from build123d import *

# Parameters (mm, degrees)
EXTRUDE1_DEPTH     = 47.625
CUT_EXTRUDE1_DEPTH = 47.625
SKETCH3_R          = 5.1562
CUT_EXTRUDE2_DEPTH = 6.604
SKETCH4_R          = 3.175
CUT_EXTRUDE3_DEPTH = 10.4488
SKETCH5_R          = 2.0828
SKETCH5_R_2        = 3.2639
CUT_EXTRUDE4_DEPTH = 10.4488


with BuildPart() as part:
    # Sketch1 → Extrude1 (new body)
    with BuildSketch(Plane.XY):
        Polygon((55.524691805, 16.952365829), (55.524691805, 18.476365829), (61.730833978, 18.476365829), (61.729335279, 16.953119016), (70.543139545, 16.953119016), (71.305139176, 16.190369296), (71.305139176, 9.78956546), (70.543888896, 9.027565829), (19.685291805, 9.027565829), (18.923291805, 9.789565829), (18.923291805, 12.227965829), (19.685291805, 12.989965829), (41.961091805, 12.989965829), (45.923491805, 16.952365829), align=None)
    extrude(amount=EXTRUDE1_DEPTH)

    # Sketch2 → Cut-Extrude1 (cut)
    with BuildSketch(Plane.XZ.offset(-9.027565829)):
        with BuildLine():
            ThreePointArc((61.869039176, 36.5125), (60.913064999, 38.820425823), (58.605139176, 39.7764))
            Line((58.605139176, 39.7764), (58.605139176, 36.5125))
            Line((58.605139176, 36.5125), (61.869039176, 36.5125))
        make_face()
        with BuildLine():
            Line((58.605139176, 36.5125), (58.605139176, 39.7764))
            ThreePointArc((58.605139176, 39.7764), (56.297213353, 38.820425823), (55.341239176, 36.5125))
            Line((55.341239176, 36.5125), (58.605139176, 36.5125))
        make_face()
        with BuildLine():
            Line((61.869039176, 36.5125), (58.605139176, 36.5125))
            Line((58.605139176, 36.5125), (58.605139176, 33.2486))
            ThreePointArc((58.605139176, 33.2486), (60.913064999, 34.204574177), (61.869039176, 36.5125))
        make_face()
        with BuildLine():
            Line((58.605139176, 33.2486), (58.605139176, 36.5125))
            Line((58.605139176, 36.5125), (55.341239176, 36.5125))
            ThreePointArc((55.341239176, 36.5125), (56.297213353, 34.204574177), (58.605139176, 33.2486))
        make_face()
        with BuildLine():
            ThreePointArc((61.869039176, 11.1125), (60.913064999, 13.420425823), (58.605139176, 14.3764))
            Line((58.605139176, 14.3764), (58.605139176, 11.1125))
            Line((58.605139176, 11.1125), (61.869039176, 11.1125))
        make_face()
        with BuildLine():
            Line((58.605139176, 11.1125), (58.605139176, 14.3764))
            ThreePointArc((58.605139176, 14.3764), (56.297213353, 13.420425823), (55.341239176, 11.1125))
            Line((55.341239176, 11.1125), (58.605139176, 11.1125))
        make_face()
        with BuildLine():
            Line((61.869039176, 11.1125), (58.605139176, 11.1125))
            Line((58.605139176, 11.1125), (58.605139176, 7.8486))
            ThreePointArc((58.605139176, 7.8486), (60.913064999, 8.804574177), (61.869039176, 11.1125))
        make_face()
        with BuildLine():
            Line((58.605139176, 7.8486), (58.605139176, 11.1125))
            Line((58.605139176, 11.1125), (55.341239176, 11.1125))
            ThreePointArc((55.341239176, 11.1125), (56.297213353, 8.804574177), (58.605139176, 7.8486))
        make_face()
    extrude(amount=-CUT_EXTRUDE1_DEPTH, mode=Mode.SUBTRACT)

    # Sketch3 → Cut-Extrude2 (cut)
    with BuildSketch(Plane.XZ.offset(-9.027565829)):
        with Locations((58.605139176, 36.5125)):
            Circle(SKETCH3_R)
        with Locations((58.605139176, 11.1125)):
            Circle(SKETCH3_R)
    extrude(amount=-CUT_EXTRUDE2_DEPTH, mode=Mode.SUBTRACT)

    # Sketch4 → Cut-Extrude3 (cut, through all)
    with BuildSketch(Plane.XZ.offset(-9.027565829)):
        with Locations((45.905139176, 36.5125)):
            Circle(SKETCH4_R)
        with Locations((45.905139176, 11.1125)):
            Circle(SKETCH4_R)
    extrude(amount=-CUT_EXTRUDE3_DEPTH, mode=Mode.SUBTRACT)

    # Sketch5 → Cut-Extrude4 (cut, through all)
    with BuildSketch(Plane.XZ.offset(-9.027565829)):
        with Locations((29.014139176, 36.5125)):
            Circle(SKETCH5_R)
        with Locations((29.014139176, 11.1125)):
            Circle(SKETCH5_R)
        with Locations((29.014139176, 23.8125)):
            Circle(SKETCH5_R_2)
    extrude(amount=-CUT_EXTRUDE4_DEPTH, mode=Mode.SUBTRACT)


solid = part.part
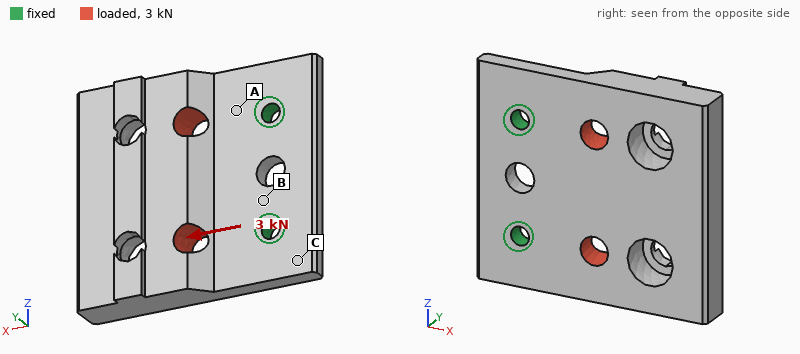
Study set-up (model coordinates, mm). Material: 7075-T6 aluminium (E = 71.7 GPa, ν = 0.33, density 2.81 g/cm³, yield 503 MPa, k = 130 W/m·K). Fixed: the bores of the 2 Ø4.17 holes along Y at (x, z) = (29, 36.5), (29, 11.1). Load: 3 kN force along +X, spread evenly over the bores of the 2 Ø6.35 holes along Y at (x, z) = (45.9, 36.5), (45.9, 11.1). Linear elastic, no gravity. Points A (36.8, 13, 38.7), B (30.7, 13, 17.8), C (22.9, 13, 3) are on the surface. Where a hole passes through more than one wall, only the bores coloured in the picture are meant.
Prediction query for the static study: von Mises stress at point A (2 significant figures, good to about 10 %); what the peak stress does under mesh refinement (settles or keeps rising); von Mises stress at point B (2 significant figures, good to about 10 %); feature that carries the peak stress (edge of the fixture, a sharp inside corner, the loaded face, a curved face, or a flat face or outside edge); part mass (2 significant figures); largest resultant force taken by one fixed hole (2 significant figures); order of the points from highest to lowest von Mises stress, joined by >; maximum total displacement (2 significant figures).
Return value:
59 MPa
keeps rising
39 MPa
edge of the fixture
38 g
1.5 kN
A > B > C
0.15 mm
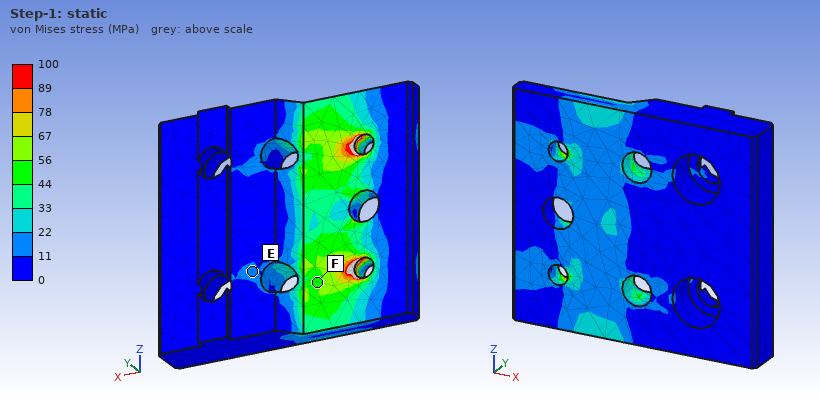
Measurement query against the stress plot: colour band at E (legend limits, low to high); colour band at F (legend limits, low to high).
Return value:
11 to 22 MPa
44 to 56 MPa
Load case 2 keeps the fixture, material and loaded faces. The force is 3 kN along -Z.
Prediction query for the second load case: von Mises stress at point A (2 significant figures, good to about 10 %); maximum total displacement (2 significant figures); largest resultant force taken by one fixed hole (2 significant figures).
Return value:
30 MPa
38 µm
2.3 kN
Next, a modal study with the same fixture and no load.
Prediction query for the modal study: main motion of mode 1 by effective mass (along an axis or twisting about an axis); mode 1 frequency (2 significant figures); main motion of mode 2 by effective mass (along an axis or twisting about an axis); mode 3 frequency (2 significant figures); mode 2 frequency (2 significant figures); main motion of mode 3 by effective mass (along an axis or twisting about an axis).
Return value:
along Y
1400 Hz
twisting about X
7900 Hz
4300 Hz
along Z
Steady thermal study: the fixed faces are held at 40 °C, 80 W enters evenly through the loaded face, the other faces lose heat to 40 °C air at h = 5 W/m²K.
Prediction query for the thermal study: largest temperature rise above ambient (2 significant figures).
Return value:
69 K
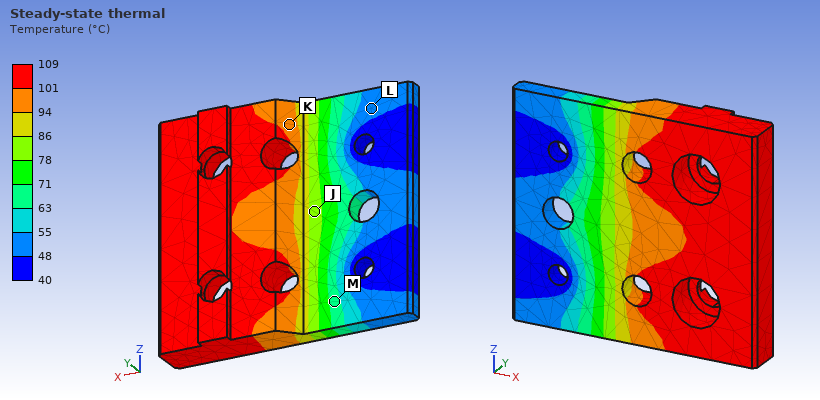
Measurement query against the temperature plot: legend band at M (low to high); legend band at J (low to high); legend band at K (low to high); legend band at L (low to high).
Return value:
63 to 71 °C
78 to 86 °C
94 to 101 °C
48 to 55 °C
